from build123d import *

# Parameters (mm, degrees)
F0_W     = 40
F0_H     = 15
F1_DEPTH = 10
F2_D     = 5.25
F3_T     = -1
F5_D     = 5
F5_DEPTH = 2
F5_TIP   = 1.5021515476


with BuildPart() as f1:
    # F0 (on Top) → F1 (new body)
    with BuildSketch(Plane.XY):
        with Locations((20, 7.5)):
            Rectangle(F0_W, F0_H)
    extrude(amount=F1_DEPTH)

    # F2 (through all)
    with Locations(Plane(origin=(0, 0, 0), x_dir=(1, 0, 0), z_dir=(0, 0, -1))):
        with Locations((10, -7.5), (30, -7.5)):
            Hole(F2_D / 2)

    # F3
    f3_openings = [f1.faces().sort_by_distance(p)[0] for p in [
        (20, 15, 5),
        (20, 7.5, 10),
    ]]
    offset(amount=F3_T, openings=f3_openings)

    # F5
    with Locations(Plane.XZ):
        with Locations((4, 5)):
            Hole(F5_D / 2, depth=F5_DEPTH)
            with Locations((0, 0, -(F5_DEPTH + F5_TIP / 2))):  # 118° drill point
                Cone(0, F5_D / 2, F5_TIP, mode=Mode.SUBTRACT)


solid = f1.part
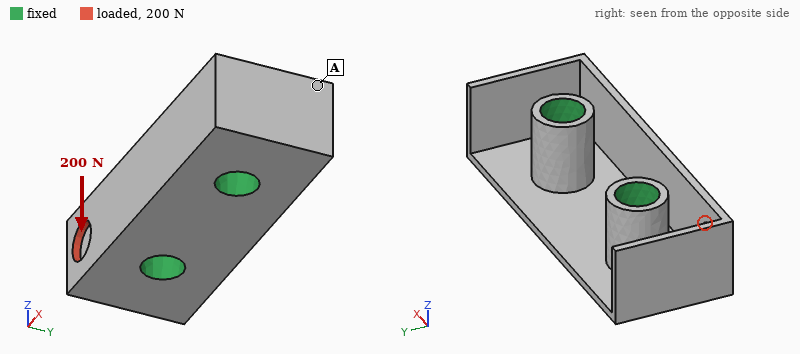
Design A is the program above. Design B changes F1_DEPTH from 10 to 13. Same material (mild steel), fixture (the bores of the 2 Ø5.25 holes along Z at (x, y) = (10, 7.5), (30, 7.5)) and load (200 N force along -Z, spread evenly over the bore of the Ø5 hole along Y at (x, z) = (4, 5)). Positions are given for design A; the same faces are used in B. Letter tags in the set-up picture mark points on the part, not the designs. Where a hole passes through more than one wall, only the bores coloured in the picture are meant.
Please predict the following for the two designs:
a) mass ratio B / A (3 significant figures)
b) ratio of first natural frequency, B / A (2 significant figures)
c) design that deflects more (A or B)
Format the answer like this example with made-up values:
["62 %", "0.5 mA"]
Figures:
["1.21", "0.70", "B"]
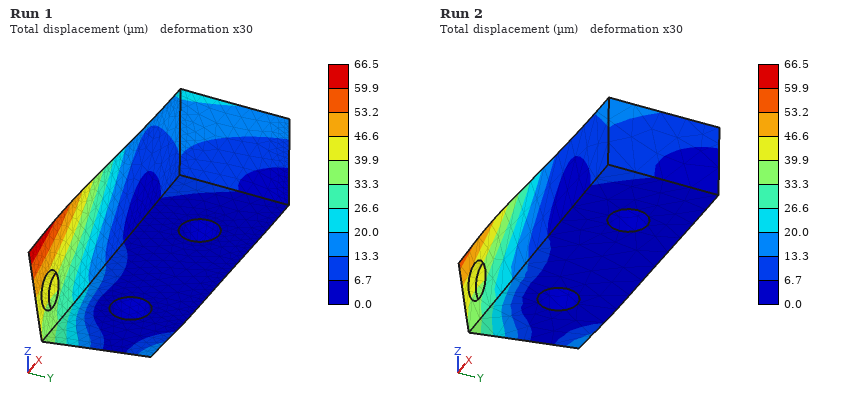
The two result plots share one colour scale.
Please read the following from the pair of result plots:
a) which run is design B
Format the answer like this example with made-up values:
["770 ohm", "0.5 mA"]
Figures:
["Run 1"]
